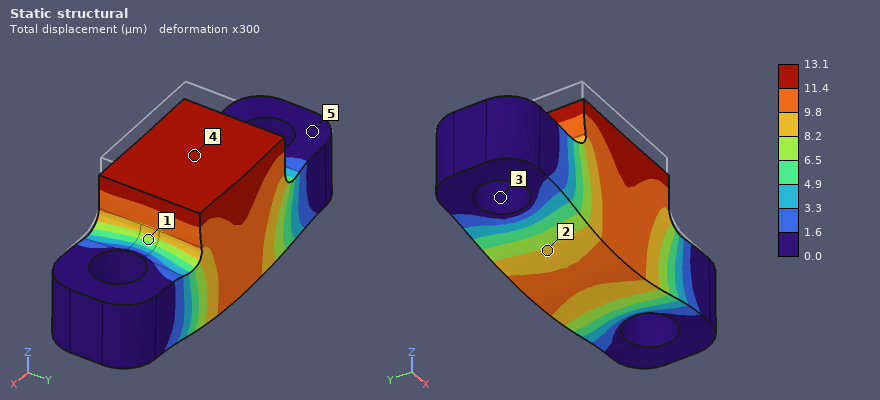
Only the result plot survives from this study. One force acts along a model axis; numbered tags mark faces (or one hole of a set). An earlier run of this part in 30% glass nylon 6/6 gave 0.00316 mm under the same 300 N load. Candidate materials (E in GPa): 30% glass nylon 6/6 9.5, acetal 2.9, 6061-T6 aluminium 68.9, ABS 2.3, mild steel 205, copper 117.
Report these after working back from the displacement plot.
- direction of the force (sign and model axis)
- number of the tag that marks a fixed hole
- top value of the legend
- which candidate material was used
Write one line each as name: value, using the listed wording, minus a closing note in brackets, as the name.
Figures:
direction of the force: -Z
number of the tag that marks a fixed hole: 3
top value of the legend: 13.1 µm
which candidate material was used: ABS
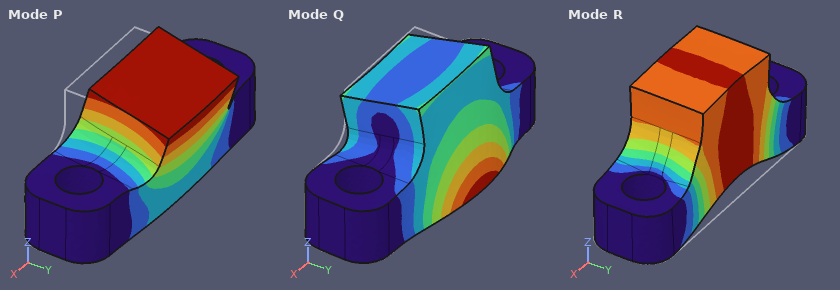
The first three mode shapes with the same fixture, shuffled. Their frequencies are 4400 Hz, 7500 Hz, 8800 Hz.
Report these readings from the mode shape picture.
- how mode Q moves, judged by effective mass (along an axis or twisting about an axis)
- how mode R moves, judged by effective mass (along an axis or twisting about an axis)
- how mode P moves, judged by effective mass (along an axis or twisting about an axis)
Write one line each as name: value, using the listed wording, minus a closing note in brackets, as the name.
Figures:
how mode Q moves, judged by effective mass: along Y
how mode R moves, judged by effective mass: along Z
how mode P moves, judged by effective mass: along Y
